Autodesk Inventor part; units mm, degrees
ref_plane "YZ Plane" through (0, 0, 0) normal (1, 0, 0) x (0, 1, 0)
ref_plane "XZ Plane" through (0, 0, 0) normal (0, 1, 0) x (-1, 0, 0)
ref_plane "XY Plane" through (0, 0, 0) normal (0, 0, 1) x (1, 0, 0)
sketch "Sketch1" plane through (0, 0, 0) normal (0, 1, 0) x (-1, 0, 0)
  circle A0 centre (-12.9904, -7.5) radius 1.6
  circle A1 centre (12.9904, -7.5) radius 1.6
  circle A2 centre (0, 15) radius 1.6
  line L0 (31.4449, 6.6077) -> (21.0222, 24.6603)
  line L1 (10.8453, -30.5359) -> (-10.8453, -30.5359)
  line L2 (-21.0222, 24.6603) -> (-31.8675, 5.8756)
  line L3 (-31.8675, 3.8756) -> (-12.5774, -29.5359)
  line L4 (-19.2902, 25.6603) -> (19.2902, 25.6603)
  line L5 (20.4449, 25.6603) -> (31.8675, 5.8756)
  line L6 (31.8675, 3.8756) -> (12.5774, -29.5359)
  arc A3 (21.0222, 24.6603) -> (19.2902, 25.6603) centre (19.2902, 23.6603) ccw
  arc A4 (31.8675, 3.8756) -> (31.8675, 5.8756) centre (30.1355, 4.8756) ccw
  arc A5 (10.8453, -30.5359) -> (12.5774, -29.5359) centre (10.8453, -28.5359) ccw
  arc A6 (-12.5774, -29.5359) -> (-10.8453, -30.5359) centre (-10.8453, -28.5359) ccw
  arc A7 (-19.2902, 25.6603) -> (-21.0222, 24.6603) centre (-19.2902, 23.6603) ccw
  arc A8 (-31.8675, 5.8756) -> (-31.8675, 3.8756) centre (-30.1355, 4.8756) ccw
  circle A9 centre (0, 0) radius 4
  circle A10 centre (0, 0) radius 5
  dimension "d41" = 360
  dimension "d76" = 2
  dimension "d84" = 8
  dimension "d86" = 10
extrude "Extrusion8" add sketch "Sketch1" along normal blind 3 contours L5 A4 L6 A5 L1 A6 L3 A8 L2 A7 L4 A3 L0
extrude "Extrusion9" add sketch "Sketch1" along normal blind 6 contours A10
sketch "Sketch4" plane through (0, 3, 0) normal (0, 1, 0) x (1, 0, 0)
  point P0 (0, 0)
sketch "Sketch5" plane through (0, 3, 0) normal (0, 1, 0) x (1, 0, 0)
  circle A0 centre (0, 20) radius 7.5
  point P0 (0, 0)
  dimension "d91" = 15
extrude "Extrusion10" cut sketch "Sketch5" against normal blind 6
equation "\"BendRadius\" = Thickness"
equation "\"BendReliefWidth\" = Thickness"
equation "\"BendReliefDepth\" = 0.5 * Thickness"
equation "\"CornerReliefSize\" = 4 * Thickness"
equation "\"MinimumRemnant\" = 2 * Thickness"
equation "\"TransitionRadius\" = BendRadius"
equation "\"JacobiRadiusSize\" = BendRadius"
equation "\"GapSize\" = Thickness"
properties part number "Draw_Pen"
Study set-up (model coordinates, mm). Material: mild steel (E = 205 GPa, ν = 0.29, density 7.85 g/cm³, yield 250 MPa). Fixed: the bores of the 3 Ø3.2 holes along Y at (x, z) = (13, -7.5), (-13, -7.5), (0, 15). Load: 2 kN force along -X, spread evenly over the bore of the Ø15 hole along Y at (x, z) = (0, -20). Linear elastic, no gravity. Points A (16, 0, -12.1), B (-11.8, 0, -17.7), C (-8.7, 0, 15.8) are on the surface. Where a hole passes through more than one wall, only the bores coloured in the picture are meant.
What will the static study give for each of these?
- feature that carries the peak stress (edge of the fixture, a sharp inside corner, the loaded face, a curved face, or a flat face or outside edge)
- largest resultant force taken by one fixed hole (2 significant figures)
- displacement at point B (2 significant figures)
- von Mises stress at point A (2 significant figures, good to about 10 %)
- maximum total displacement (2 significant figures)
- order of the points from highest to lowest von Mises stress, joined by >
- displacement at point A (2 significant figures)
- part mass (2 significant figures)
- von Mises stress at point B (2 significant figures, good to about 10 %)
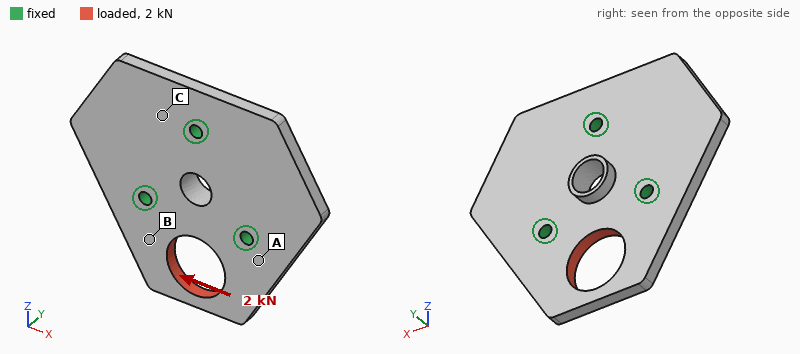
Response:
edge of the fixture
1.3 kN
4.0 µm
21 MPa
11 µm
B > A > C
1.8 µm
58 g
30 MPa
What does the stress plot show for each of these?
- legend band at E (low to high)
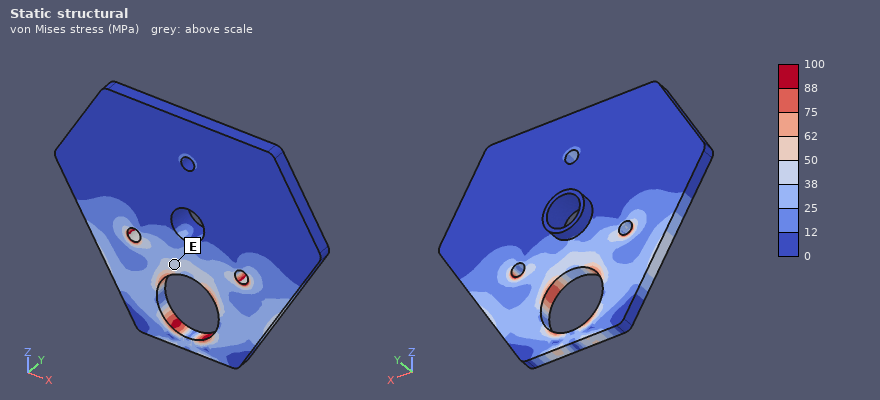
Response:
38 to 50 MPa
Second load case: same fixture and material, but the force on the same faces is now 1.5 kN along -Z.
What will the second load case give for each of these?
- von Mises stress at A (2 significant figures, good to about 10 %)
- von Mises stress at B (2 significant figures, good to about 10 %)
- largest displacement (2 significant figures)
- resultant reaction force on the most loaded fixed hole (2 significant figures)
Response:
9.9 MPa
21 MPa
4.6 µm
710 N
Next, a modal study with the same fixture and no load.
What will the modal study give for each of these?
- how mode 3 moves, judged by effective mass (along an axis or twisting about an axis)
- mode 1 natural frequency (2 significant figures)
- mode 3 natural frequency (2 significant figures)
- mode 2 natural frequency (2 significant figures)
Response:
along Y
4900 Hz
5600 Hz
5000 Hz
